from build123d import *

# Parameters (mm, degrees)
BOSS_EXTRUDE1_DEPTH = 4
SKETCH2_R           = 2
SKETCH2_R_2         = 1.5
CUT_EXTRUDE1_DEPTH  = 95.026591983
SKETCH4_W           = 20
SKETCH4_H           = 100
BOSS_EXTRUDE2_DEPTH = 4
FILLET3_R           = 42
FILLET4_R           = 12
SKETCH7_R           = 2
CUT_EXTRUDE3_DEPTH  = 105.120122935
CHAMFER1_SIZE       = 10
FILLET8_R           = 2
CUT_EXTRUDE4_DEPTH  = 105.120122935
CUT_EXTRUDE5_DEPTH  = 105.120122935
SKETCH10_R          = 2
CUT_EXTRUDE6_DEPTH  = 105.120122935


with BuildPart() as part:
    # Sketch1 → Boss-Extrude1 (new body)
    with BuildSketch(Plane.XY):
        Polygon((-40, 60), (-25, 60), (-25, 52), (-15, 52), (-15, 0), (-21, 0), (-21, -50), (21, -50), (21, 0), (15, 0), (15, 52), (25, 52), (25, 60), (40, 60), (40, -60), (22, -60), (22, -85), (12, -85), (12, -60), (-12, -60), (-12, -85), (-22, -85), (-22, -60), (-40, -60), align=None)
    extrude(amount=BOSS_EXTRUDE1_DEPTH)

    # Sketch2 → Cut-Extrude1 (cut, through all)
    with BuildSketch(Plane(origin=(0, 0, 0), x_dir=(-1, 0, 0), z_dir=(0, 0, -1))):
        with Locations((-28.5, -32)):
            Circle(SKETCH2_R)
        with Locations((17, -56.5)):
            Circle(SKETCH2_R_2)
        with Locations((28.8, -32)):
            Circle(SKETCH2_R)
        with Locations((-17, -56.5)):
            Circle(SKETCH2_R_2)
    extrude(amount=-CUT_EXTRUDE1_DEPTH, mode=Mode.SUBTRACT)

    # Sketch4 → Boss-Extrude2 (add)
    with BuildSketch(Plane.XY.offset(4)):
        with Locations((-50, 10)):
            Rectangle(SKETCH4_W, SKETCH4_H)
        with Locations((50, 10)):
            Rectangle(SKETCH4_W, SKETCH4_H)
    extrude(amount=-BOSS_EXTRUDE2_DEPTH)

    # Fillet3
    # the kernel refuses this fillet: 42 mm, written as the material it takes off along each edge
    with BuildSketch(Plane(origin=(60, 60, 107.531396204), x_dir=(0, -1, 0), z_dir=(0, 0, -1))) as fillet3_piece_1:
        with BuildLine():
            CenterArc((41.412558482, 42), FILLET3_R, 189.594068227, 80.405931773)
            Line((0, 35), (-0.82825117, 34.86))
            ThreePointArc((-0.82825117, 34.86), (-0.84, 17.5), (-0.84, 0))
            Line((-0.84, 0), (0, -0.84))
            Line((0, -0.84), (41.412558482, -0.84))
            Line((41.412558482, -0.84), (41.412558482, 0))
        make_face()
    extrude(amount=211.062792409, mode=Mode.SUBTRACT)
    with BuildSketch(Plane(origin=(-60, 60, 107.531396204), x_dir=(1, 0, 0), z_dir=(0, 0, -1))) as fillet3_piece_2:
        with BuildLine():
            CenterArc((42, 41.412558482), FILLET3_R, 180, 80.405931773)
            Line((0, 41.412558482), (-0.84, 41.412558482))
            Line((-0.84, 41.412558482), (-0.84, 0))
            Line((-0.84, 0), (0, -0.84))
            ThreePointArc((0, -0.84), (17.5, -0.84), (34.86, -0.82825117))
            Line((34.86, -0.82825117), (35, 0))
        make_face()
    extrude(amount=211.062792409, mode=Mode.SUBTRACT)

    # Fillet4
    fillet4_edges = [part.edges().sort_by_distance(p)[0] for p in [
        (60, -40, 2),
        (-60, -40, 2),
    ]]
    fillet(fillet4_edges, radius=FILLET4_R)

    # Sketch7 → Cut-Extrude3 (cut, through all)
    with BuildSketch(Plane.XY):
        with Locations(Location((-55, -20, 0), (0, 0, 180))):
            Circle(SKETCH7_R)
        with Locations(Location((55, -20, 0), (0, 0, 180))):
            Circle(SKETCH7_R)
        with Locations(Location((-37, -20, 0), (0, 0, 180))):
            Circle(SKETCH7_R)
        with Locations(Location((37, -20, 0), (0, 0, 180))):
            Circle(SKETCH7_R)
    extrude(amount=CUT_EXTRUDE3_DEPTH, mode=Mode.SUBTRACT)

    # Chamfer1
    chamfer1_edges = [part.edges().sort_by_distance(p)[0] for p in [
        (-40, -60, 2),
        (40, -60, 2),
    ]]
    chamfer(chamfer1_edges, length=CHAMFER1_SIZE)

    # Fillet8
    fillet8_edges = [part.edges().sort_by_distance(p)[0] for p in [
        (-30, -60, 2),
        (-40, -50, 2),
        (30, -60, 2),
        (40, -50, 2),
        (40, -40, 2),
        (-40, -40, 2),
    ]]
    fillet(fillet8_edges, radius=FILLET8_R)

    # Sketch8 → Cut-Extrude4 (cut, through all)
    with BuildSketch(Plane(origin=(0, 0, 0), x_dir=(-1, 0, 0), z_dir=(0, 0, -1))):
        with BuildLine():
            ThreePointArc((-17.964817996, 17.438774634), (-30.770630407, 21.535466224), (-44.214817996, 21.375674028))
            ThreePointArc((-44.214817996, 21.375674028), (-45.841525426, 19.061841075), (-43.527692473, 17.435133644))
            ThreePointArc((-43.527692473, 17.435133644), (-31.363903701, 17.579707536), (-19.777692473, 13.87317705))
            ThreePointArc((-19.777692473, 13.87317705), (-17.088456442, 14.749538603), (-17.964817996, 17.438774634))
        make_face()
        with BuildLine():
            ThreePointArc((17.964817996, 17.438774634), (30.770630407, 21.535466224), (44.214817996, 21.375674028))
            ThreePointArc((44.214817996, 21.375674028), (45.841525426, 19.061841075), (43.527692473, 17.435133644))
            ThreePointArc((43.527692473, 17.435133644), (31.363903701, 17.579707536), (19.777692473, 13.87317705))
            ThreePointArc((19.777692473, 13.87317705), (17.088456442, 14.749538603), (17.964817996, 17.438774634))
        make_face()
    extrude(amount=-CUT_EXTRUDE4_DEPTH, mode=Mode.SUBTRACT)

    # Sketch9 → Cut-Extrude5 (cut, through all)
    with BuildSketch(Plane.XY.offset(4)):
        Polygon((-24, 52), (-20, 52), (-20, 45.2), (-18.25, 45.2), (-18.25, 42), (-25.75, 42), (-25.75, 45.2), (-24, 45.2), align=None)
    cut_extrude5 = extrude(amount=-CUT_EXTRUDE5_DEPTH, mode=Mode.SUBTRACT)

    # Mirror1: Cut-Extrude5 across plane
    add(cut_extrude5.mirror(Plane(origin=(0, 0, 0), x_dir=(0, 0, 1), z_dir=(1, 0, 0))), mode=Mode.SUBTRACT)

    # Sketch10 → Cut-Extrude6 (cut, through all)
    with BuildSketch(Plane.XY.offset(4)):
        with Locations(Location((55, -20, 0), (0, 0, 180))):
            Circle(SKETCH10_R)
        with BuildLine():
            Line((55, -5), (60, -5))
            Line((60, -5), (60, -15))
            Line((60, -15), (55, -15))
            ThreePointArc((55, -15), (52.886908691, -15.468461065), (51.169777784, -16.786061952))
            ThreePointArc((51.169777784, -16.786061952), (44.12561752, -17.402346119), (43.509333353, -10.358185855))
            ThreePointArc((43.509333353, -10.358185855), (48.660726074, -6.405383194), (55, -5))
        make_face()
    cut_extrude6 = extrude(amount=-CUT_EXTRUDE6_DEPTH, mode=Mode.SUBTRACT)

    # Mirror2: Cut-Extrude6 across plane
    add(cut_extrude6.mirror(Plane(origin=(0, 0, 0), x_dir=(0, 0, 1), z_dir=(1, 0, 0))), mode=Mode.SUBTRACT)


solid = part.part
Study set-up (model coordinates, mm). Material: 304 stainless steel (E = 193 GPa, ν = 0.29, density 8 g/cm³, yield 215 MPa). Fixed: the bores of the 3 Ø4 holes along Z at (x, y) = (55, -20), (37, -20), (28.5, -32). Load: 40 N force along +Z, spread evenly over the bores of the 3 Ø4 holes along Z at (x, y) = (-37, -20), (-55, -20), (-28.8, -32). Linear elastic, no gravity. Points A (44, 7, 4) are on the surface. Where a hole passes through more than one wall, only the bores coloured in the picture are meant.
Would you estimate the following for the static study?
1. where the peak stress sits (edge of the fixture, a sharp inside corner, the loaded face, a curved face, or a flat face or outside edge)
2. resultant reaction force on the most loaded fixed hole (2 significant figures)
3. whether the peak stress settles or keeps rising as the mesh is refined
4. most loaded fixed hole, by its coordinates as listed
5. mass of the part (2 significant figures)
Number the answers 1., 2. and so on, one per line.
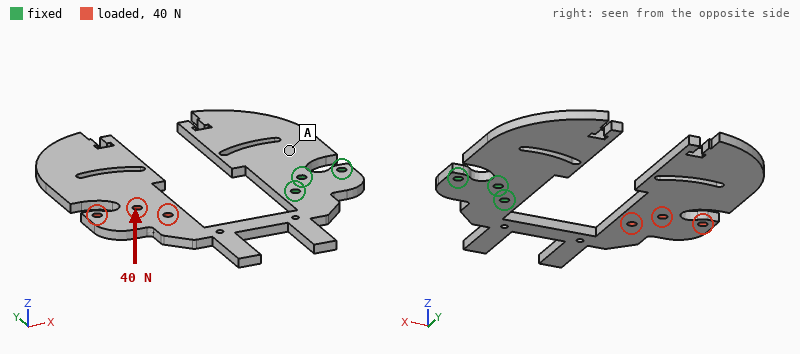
1. a sharp inside corner
2. 67 N
3. keeps rising
4. (28.5, -32)
5. 270 g
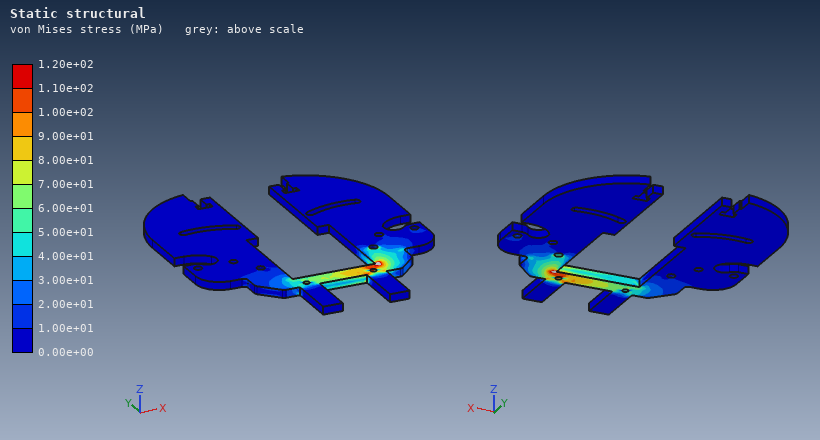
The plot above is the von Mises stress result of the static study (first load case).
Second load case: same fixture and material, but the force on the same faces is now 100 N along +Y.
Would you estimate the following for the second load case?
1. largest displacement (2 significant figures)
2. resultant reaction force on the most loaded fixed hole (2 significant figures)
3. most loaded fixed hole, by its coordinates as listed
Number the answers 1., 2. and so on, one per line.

1. 0.41 mm
2. 430 N
3. (28.5, -32)
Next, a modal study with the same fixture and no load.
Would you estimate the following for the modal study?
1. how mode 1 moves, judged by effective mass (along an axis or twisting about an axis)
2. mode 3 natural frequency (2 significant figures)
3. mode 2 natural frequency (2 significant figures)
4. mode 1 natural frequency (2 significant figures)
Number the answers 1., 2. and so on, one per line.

1. along Z
2. 260 Hz
3. 210 Hz
4. 79 Hz
